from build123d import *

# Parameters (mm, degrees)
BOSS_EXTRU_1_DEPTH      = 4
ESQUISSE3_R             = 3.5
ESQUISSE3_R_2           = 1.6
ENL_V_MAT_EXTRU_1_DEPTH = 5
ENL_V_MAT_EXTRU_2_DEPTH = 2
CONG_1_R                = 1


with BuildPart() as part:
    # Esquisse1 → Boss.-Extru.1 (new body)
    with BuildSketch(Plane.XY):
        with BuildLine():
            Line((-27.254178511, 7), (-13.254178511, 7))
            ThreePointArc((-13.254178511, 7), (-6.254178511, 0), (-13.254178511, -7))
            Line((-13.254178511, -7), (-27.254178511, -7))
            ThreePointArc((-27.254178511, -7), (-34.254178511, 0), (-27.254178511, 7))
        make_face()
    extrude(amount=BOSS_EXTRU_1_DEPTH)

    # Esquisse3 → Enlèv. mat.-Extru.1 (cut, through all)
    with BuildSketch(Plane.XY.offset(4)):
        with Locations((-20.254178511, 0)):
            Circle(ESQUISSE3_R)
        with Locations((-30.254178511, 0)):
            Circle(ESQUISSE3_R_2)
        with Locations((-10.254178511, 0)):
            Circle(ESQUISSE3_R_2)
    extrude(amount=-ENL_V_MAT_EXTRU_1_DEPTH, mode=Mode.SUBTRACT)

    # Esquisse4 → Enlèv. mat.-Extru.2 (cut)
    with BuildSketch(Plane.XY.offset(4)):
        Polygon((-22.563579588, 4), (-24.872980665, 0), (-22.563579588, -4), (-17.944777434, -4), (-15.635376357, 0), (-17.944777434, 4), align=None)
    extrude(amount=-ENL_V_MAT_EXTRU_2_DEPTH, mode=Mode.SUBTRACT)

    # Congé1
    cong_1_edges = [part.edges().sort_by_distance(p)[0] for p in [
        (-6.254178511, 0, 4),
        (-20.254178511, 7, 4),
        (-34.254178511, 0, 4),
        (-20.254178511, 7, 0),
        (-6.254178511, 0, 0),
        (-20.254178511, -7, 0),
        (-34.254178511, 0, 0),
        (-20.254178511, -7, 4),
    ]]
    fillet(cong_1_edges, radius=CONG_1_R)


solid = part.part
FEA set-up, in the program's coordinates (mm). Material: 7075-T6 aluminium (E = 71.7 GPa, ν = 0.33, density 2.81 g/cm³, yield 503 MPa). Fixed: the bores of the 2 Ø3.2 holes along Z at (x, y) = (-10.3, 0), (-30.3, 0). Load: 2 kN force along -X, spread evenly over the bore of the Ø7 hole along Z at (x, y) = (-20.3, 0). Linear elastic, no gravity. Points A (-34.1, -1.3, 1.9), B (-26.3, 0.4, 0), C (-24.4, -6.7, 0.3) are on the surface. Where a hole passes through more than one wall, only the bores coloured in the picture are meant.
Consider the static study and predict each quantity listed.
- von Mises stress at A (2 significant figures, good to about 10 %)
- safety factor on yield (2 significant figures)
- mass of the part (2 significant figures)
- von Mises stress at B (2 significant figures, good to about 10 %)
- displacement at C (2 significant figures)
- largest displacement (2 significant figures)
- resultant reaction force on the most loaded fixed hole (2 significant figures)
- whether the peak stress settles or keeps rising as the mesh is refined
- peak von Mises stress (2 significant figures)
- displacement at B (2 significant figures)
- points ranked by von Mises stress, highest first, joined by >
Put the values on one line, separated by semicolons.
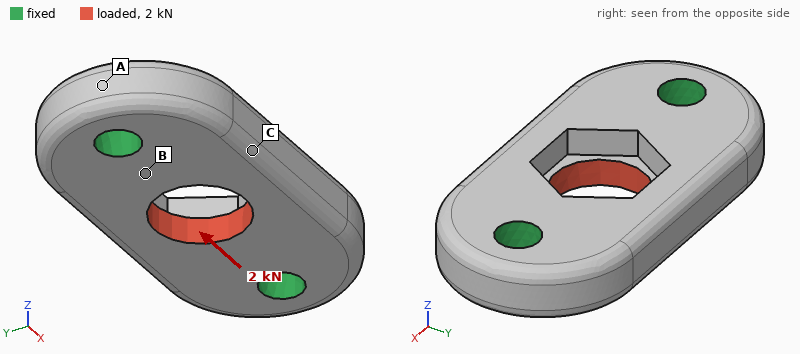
15 MPa; 5.4; 3.1 g; 59 MPa; 3.2 µm; 5.2 µm; 1.0 kN; settles; 93 MPa; 2.0 µm; B > A > C
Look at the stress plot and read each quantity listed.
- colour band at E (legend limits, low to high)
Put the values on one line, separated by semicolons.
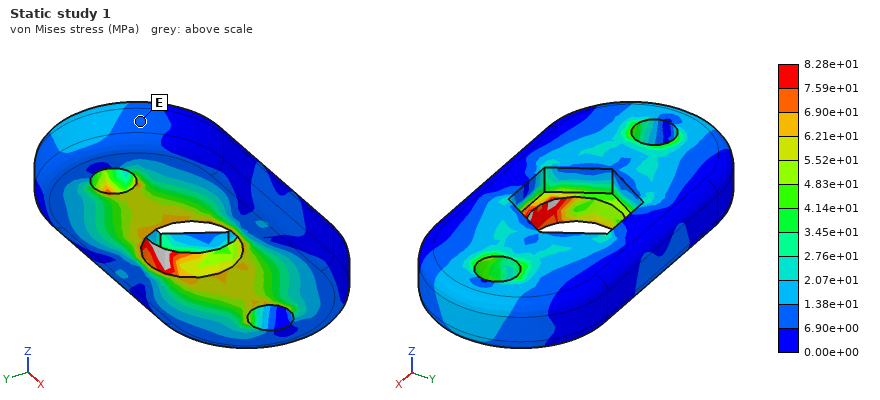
6.90e+00 to 1.38e+01 MPa
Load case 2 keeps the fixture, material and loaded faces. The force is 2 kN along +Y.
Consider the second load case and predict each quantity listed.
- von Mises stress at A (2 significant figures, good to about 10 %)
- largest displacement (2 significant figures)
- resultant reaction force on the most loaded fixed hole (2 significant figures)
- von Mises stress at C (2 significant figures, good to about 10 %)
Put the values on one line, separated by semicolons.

8.7 MPa; 14 µm; 1.0 kN; 29 MPa
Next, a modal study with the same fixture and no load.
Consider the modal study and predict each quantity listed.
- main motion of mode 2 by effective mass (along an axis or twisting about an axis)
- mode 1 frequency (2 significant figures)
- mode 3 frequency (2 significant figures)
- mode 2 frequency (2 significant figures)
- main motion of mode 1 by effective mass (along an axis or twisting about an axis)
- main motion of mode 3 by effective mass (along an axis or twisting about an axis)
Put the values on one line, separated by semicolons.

along Z; 40 kHz; 69 kHz; 42 kHz; twisting about X; along Y
